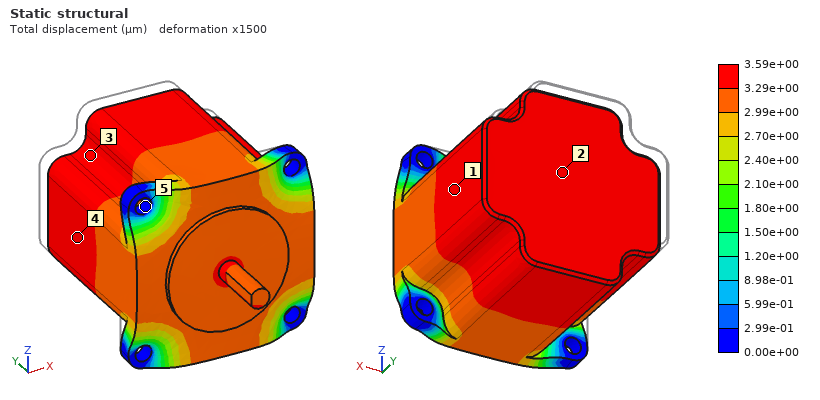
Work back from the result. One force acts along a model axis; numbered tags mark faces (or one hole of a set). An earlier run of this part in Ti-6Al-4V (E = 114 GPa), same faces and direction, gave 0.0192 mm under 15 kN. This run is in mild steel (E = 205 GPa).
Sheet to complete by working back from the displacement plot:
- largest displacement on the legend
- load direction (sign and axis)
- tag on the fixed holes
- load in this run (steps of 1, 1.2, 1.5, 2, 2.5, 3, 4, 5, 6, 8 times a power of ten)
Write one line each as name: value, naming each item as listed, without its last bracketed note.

largest displacement on the legend: 3.59e+00 µm
load direction: -Y
tag on the fixed holes: 5
load in this run: 5 kN
